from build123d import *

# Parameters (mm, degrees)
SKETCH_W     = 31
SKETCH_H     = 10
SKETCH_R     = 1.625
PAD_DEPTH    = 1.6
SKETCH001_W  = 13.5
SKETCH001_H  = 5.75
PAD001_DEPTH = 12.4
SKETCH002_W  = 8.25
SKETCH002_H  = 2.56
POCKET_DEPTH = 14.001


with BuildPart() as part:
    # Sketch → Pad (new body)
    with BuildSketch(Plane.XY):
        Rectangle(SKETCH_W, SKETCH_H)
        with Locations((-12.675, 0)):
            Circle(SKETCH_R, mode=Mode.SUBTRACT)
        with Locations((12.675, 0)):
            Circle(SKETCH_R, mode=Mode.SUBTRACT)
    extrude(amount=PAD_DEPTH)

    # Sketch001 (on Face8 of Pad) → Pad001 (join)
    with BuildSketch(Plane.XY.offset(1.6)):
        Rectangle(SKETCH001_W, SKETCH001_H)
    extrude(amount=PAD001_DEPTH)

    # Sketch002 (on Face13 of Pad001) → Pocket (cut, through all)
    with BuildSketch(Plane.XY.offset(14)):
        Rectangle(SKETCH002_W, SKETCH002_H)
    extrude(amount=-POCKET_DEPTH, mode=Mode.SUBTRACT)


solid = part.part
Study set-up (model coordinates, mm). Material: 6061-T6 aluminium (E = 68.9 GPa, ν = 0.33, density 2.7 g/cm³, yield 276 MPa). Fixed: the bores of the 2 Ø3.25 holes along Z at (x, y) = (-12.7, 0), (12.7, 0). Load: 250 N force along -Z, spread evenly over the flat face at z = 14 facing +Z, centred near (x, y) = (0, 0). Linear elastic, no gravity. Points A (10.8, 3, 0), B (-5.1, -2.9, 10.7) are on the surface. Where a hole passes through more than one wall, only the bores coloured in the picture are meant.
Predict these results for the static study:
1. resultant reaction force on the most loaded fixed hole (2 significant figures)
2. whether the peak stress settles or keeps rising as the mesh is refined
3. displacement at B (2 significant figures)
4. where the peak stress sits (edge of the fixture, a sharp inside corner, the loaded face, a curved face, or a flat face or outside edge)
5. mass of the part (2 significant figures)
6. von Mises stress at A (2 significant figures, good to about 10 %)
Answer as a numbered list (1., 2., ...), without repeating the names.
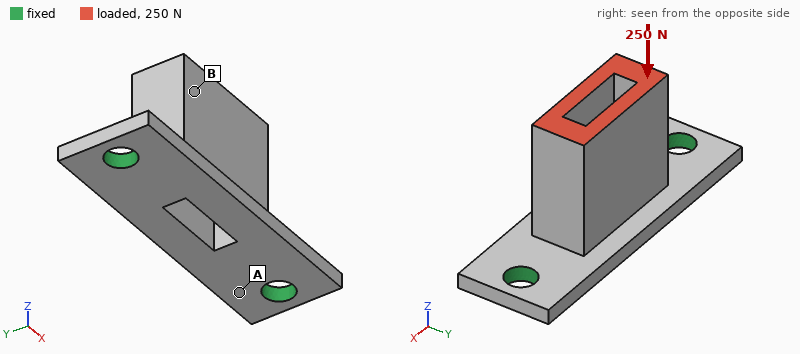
1. 140 N
2. keeps rising
3. 14 µm
4. edge of the fixture
5. 3.1 g
6. 34 MPa
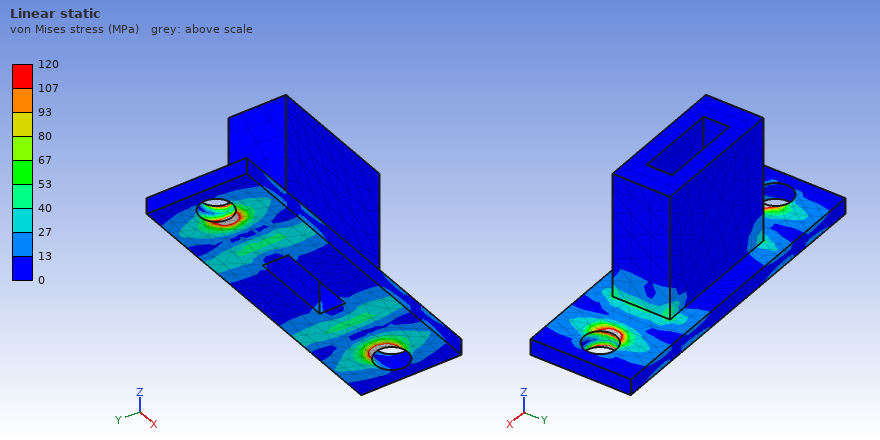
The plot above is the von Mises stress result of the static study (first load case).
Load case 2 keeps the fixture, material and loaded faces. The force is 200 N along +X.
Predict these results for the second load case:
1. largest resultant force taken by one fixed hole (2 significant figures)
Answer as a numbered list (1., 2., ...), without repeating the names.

1. 180 N
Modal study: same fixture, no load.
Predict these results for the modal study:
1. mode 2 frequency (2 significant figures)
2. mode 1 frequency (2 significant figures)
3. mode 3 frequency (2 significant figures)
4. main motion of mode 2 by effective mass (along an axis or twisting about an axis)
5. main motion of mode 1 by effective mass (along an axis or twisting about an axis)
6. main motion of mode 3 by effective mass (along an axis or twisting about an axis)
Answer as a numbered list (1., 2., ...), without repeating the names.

1. 14 kHz
2. 5300 Hz
3. 15 kHz
4. along Z
5. along Y
6. along X
